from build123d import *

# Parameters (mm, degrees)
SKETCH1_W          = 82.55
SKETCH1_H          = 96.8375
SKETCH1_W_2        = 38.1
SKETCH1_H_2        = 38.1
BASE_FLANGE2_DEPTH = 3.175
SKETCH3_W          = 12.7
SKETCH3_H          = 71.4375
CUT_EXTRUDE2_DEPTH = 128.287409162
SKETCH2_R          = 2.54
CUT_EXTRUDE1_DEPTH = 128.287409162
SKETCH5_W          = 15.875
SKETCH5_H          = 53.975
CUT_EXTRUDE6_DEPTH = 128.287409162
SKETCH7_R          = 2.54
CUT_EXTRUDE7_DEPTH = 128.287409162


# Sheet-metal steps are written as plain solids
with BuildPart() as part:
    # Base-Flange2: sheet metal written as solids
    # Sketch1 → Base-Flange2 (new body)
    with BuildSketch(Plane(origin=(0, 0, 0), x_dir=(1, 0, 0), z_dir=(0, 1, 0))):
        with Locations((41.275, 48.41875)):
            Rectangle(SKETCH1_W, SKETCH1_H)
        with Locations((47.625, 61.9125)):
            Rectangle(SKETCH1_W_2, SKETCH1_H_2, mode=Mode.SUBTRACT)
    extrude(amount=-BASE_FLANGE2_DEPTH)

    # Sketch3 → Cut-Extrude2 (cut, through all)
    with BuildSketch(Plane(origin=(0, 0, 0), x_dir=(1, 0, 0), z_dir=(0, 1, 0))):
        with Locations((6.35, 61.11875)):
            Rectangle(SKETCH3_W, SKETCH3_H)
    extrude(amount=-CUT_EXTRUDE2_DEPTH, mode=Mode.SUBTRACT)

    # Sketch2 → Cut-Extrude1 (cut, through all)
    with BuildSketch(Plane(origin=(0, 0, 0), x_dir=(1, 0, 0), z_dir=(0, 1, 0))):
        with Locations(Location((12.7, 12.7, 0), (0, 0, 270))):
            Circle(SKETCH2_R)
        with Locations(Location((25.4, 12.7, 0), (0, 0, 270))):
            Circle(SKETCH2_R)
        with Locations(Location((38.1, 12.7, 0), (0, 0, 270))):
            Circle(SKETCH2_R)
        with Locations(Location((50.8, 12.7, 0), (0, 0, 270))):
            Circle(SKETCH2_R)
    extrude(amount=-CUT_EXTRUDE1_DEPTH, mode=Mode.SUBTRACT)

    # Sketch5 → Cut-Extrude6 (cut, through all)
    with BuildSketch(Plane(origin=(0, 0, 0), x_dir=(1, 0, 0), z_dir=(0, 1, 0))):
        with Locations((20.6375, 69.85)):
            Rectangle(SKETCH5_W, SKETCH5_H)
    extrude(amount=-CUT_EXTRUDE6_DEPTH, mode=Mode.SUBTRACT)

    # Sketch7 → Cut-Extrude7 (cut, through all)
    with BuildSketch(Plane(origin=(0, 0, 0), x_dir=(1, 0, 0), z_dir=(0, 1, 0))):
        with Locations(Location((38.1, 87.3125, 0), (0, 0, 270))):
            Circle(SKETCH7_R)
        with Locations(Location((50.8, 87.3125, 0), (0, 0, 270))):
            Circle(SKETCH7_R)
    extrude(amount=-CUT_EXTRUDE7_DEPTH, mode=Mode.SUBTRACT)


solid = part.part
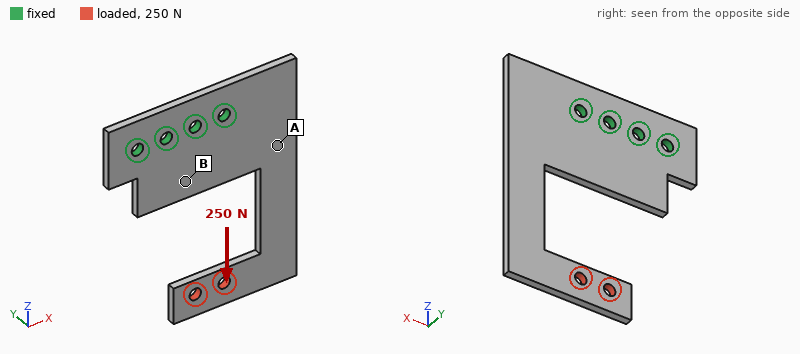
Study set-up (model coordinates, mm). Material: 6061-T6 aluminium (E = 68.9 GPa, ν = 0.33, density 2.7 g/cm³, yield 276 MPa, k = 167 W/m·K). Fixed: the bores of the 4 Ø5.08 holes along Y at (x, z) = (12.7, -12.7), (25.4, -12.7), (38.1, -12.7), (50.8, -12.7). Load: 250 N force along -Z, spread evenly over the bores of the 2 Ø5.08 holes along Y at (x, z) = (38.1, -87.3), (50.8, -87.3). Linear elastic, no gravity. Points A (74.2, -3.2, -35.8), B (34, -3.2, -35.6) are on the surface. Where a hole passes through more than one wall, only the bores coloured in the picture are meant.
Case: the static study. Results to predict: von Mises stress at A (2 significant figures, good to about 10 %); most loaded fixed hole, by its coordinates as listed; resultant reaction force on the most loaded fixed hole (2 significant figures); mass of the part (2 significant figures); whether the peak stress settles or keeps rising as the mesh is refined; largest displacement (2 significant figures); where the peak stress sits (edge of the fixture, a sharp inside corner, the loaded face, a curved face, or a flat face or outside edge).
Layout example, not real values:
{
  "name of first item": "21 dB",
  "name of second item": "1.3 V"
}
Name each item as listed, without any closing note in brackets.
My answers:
{
  "von Mises stress at A": "15 MPa",
  "most loaded fixed hole, by its coordinates as listed": "(50.8, -12.7)",
  "resultant reaction force on the most loaded fixed hole": "170 N",
  "mass of the part": "40 g",
  "whether the peak stress settles or keeps rising as the mesh is refined": "keeps rising",
  "largest displacement": "0.37 mm",
  "where the peak stress sits": "a sharp inside corner"
}
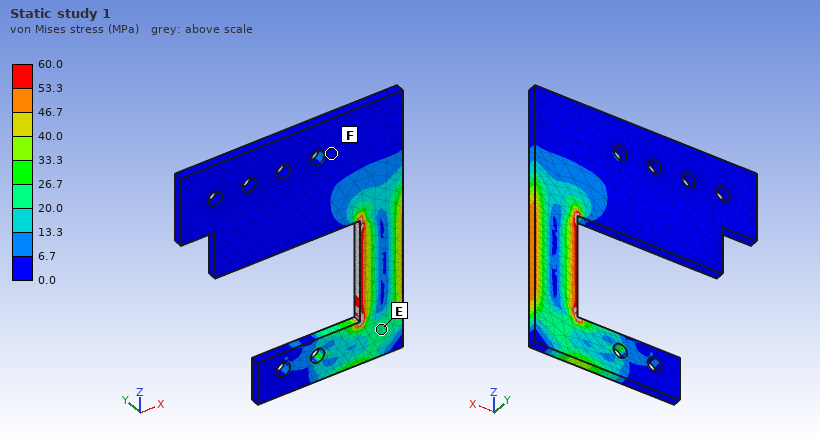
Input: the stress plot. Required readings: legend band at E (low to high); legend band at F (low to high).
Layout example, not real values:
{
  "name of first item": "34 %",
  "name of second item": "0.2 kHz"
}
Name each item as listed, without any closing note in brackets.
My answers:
{
  "legend band at E": "20.0 to 26.7 MPa",
  "legend band at F": "0.0 to 6.7 MPa"
}
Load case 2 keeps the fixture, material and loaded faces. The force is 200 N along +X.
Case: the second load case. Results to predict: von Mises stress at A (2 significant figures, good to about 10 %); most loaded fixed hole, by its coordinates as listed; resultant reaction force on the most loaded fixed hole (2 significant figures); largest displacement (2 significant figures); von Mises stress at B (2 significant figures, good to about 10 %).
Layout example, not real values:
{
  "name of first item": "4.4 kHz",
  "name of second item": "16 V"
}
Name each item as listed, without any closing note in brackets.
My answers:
{
  "von Mises stress at A": "18 MPa",
  "most loaded fixed hole, by its coordinates as listed": "(50.8, -12.7)",
  "resultant reaction force on the most loaded fixed hole": "440 N",
  "largest displacement": "0.28 mm",
  "von Mises stress at B": "6.6 MPa"
}
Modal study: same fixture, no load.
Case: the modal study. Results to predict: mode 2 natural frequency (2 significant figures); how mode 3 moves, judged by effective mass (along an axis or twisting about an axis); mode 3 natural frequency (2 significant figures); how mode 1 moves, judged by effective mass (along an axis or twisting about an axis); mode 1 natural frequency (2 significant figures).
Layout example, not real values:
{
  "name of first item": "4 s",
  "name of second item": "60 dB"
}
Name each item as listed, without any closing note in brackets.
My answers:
{
  "mode 2 natural frequency": "750 Hz",
  "how mode 3 moves, judged by effective mass": "along X",
  "mode 3 natural frequency": "1600 Hz",
  "how mode 1 moves, judged by effective mass": "along Y",
  "mode 1 natural frequency": "300 Hz"
}
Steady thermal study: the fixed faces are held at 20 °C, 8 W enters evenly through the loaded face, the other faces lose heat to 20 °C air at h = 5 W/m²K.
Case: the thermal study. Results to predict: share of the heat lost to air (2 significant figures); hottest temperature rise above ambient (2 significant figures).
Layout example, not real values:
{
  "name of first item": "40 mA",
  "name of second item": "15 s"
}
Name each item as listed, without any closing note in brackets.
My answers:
{
  "share of the heat lost to air": "13 %",
  "hottest temperature rise above ambient": "81 K"
}
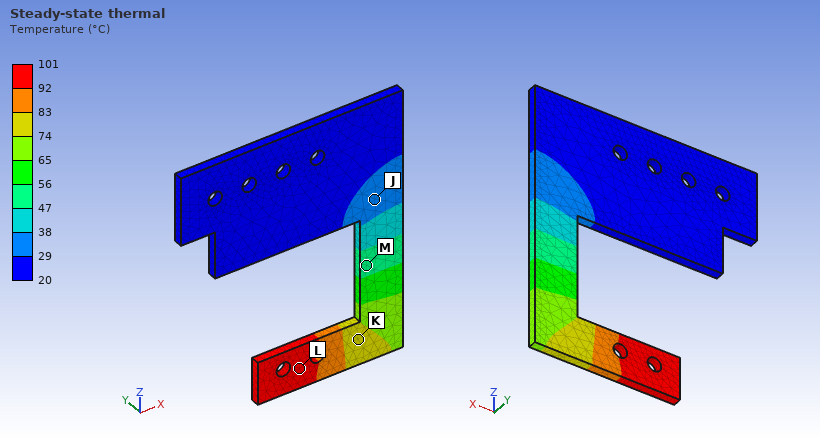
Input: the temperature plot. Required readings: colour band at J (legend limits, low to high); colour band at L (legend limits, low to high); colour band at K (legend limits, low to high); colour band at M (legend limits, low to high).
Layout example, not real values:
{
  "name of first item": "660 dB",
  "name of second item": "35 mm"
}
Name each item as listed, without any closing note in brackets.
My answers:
{
  "colour band at J": "29 to 38 °C",
  "colour band at L": "92 to 101 °C",
  "colour band at K": "74 to 83 °C",
  "colour band at M": "47 to 56 °C"
}
